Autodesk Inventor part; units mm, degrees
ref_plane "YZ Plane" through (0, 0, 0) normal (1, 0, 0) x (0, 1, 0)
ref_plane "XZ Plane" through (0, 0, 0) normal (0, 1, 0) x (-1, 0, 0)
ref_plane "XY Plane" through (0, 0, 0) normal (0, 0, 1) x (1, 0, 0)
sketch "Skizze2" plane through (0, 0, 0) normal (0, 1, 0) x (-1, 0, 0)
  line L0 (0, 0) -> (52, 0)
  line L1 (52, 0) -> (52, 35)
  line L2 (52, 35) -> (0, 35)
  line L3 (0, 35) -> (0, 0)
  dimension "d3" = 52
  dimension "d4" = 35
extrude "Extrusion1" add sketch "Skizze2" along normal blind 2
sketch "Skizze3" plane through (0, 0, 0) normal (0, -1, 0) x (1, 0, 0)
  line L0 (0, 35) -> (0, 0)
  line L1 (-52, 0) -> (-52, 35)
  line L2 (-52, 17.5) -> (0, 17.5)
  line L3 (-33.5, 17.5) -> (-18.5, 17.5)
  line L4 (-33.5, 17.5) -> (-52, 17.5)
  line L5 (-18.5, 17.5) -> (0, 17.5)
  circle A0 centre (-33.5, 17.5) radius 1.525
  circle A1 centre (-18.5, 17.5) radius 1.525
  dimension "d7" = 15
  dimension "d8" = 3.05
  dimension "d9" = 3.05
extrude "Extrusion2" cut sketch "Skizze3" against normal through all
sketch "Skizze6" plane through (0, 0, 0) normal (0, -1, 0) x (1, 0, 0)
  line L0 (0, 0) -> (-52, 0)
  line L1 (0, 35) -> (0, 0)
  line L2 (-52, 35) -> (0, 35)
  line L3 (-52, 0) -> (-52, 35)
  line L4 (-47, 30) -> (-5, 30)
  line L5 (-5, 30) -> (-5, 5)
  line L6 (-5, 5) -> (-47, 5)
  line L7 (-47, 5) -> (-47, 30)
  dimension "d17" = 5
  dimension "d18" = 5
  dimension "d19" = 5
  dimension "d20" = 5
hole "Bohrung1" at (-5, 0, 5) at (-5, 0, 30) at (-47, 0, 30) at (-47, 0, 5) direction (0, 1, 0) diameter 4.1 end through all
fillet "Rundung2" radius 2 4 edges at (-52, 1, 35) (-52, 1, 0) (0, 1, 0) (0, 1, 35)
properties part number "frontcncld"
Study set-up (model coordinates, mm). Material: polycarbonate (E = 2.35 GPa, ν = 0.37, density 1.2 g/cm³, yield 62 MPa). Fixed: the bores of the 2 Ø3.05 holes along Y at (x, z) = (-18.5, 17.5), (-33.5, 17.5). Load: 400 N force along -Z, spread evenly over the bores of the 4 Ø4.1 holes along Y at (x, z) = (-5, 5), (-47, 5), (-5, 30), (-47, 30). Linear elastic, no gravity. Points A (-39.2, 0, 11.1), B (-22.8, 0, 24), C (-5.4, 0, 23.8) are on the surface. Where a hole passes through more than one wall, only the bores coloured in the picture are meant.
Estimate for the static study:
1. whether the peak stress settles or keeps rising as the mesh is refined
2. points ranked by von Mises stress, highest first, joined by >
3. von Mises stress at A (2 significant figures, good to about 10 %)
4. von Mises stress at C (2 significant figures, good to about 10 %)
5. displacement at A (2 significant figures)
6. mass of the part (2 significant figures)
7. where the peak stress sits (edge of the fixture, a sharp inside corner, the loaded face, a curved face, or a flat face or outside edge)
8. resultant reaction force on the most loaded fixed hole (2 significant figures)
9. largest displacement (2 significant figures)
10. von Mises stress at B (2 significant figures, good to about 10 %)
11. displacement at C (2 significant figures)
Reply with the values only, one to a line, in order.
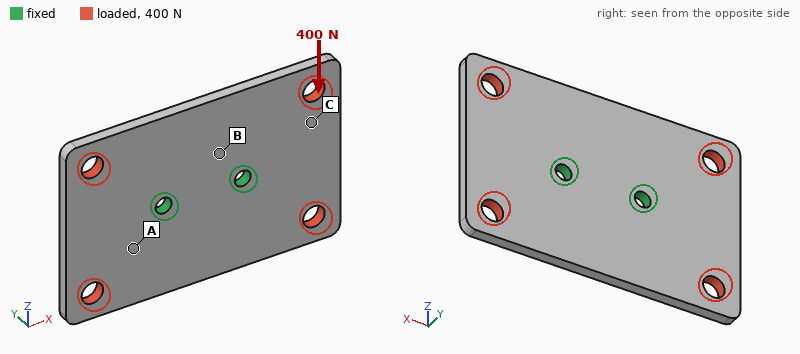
keeps rising
A > C > B
6.8 MPa
4.5 MPa
0.042 mm
4.2 g
edge of the fixture
200 N
0.12 mm
1.8 MPa
0.084 mm
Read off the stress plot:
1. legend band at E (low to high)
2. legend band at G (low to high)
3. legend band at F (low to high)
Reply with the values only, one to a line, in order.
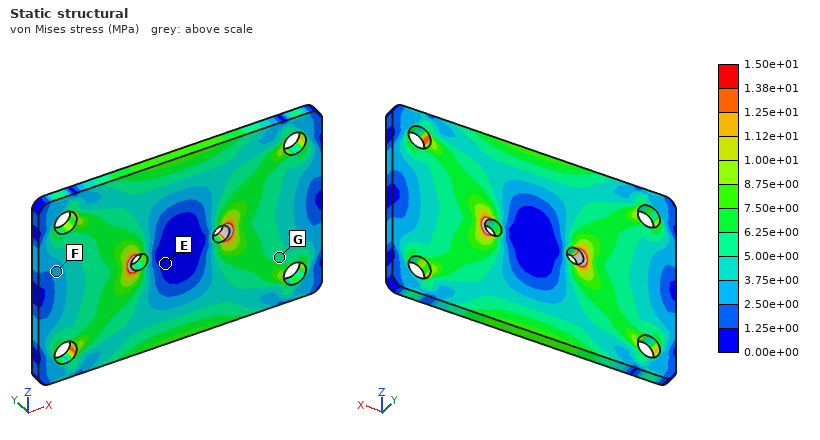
0.00e+00 to 1.25e+00 MPa
5.00e+00 to 6.25e+00 MPa
2.50e+00 to 3.75e+00 MPa
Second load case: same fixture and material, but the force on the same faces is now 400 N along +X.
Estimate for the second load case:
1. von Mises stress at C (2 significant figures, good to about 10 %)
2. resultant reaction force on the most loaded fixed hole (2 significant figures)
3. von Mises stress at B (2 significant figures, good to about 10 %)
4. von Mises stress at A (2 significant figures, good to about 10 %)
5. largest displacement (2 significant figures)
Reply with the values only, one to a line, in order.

4.0 MPa
200 N
4.2 MPa
4.3 MPa
70 µm
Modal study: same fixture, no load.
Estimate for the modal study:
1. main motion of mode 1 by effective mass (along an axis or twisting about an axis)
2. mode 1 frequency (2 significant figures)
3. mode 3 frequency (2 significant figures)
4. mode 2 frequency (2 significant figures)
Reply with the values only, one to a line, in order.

twisting about X
1100 Hz
1200 Hz
1200 Hz
